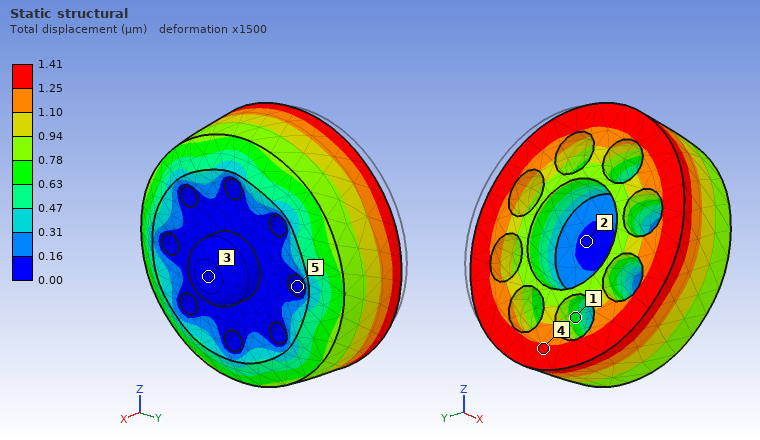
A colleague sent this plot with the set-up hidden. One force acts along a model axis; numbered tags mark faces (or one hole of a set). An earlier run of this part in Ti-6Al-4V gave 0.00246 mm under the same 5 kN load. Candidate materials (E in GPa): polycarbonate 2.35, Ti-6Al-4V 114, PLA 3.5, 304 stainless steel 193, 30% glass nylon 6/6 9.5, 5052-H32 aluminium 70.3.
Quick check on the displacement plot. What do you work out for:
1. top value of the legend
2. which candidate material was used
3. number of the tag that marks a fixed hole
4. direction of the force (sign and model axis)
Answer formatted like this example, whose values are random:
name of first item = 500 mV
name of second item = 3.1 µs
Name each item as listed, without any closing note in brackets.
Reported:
top value of the legend = 1.41 µm
which candidate material was used = 304 stainless steel
number of the tag that marks a fixed hole = 5
direction of the force = +X
